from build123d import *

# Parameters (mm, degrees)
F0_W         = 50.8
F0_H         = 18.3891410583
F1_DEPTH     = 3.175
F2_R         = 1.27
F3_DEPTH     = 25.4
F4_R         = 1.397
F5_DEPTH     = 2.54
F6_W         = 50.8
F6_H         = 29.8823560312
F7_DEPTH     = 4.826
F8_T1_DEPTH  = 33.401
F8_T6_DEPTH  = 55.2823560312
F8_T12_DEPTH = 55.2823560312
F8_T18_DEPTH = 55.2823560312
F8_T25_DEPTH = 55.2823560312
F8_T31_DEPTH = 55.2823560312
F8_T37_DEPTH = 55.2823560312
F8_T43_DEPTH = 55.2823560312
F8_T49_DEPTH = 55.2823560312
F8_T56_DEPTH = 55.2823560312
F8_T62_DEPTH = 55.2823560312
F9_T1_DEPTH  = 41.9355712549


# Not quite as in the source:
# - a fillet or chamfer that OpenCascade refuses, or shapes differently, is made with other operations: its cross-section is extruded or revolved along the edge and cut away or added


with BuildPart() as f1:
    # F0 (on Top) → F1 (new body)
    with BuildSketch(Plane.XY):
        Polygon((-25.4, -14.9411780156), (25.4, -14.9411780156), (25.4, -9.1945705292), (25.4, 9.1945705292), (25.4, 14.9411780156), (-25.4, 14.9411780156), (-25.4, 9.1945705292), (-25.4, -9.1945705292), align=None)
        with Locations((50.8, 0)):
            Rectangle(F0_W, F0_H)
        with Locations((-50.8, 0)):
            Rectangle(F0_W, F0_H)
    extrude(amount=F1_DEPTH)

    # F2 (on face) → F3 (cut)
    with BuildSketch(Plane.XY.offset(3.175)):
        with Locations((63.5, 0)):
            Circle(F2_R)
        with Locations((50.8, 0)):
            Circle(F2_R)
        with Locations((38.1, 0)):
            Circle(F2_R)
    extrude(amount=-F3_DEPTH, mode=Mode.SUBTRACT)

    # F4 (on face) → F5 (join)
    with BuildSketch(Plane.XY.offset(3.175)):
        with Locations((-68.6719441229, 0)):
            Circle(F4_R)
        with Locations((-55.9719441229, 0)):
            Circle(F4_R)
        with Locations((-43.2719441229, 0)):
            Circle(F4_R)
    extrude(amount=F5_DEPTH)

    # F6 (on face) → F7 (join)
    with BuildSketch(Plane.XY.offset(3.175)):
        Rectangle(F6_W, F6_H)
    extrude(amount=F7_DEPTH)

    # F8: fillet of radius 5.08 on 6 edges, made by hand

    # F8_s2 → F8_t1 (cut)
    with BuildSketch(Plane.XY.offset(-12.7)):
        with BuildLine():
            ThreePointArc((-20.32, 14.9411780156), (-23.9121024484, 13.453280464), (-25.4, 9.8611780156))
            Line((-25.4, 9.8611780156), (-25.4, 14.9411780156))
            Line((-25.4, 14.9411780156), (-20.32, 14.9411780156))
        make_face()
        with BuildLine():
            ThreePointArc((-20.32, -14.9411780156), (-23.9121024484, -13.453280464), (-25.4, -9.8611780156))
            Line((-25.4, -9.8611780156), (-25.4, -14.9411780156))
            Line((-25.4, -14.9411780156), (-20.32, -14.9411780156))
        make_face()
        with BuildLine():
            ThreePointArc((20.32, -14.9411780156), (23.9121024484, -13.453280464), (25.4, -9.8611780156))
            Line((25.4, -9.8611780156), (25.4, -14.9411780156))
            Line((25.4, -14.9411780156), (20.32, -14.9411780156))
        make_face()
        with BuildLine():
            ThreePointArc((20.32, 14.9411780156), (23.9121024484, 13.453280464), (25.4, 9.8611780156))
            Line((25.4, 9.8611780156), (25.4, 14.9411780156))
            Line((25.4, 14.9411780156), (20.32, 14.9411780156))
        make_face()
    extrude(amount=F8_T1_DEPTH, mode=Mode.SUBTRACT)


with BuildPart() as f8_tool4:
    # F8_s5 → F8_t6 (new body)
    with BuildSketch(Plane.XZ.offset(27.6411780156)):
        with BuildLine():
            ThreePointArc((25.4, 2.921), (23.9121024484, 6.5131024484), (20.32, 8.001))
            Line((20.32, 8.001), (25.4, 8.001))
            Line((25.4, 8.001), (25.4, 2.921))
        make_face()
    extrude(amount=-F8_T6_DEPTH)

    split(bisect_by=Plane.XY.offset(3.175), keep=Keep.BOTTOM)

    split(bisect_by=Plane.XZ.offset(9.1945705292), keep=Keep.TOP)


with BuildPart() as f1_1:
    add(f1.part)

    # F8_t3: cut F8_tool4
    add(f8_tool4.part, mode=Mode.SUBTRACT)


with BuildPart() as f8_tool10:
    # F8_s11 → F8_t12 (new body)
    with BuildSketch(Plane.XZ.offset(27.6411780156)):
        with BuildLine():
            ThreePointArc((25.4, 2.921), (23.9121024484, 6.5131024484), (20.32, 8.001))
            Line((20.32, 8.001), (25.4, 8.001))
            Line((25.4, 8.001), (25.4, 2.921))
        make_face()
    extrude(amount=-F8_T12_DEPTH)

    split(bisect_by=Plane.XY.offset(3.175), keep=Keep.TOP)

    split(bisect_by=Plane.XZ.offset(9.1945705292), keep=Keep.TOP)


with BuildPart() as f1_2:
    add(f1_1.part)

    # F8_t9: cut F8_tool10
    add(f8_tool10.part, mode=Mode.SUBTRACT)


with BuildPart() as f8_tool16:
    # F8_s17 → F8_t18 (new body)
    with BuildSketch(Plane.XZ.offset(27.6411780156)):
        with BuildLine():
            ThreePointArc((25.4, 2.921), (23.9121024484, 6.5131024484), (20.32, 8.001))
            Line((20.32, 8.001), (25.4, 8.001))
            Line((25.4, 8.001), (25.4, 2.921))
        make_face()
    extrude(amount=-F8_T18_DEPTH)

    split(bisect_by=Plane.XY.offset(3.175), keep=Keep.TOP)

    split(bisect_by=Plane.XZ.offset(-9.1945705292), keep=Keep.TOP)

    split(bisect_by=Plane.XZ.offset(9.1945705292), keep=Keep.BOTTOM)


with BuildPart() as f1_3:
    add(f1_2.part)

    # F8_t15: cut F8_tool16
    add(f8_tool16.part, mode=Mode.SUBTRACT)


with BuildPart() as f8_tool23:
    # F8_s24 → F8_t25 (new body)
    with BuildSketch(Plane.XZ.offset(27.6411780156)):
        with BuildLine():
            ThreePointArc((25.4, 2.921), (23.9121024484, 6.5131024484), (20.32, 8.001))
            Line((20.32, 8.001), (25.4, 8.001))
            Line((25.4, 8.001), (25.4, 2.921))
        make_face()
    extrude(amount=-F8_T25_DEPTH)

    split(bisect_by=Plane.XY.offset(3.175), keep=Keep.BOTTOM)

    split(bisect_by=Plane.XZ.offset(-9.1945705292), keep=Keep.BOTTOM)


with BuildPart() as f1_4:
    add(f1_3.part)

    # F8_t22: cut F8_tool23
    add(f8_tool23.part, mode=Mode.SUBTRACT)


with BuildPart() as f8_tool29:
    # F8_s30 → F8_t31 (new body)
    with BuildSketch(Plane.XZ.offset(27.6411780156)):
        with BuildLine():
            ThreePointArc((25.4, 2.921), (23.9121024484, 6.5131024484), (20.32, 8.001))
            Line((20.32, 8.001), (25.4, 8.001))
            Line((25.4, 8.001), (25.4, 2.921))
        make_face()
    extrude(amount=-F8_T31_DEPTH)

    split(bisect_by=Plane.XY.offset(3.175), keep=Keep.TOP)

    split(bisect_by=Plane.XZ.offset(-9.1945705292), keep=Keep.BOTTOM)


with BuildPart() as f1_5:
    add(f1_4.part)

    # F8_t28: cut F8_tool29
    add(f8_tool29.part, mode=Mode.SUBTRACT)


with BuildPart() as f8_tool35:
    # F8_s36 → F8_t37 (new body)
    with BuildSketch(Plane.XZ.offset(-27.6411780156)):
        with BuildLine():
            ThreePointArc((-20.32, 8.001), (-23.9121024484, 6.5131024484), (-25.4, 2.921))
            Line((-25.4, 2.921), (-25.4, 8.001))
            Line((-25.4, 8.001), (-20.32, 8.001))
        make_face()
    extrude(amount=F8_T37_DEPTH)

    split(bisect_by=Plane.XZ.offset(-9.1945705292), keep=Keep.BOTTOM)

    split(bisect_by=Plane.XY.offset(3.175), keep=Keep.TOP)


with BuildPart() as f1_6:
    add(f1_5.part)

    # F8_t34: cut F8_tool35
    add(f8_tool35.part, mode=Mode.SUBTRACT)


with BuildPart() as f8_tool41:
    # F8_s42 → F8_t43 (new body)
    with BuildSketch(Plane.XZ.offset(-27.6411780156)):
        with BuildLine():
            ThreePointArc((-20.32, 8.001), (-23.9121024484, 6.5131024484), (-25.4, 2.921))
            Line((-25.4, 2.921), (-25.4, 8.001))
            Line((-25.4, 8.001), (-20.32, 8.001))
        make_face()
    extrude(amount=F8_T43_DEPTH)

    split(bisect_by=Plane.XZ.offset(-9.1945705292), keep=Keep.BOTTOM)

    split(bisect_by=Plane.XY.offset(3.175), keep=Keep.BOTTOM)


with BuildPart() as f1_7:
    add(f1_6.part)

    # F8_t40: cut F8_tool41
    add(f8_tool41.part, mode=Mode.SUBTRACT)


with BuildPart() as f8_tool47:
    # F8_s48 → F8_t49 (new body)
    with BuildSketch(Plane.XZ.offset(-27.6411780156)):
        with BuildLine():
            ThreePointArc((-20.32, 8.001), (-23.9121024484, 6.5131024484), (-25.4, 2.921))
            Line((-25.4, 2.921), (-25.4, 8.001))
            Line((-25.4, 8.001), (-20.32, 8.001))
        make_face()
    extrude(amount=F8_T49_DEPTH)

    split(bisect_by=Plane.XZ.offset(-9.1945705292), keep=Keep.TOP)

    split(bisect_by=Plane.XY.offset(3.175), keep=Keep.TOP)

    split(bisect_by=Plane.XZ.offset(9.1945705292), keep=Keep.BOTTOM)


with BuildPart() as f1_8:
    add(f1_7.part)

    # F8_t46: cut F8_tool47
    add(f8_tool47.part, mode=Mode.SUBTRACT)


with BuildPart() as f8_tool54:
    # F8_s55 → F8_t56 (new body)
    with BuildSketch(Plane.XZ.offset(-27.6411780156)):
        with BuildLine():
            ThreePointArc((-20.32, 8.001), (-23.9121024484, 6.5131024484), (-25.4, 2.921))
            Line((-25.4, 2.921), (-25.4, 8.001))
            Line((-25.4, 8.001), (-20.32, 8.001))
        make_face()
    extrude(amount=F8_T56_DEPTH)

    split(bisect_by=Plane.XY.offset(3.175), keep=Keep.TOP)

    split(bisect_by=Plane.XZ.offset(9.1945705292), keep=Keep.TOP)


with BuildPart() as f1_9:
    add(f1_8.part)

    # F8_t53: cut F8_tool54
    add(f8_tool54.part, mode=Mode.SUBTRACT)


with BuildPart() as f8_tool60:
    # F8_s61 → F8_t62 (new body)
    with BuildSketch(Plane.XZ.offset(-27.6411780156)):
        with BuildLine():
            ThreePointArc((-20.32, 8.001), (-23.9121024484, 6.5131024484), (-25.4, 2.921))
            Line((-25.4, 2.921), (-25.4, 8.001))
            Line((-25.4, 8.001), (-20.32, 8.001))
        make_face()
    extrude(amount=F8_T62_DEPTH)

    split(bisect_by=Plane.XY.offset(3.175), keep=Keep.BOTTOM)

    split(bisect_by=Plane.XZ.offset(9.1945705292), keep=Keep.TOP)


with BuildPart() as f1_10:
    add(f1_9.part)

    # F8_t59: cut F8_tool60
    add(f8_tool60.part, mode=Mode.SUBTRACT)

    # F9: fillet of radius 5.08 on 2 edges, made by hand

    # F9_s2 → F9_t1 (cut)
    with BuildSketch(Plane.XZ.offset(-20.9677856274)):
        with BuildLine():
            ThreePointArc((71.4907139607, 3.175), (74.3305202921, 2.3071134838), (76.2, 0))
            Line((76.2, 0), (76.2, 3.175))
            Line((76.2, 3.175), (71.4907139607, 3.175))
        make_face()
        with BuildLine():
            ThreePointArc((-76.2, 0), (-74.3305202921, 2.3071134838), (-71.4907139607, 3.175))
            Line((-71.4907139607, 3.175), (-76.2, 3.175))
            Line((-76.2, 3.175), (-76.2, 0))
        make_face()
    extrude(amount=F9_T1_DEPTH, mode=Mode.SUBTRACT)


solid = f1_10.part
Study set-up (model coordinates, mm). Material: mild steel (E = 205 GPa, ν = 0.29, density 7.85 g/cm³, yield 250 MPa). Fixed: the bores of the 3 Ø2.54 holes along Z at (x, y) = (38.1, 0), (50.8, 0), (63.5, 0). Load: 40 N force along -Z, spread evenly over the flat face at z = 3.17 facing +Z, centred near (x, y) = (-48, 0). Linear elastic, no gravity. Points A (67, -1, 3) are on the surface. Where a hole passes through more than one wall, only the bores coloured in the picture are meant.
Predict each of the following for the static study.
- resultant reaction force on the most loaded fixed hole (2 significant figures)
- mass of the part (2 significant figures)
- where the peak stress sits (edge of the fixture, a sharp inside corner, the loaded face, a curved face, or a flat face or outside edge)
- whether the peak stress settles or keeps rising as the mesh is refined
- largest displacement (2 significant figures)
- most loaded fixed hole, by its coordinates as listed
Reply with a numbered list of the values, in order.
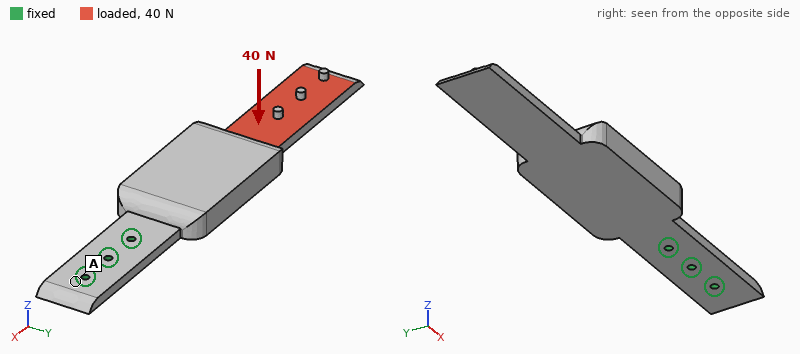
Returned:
1. 150 N
2. 140 g
3. edge of the fixture
4. keeps rising
5. 0.58 mm
6. (38.1, 0)
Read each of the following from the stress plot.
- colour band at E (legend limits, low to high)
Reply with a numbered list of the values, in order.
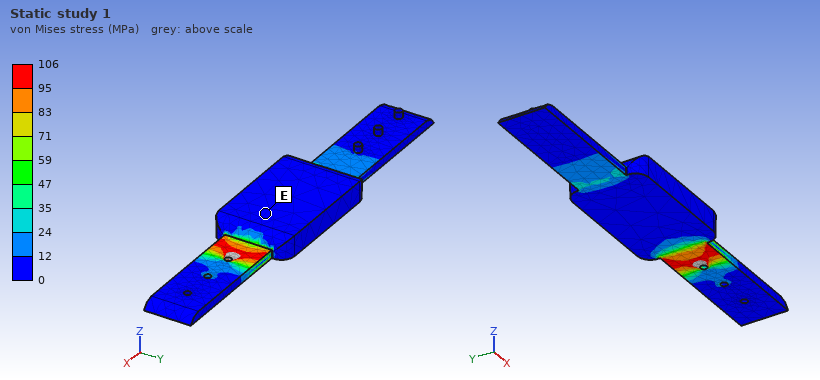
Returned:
1. 0 to 12 MPa
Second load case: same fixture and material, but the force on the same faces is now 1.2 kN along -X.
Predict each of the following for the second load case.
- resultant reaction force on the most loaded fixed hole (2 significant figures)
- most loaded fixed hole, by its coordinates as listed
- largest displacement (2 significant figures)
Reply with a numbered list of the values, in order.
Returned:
1. 890 N
2. (38.1, 0)
3. 0.43 mm
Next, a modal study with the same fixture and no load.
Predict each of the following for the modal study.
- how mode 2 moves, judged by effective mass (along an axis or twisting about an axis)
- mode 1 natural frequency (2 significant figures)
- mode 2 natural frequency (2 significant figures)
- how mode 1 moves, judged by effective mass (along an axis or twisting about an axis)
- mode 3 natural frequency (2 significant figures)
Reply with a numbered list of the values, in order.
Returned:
1. along Y
2. 250 Hz
3. 1000 Hz
4. along Z
5. 1300 Hz
